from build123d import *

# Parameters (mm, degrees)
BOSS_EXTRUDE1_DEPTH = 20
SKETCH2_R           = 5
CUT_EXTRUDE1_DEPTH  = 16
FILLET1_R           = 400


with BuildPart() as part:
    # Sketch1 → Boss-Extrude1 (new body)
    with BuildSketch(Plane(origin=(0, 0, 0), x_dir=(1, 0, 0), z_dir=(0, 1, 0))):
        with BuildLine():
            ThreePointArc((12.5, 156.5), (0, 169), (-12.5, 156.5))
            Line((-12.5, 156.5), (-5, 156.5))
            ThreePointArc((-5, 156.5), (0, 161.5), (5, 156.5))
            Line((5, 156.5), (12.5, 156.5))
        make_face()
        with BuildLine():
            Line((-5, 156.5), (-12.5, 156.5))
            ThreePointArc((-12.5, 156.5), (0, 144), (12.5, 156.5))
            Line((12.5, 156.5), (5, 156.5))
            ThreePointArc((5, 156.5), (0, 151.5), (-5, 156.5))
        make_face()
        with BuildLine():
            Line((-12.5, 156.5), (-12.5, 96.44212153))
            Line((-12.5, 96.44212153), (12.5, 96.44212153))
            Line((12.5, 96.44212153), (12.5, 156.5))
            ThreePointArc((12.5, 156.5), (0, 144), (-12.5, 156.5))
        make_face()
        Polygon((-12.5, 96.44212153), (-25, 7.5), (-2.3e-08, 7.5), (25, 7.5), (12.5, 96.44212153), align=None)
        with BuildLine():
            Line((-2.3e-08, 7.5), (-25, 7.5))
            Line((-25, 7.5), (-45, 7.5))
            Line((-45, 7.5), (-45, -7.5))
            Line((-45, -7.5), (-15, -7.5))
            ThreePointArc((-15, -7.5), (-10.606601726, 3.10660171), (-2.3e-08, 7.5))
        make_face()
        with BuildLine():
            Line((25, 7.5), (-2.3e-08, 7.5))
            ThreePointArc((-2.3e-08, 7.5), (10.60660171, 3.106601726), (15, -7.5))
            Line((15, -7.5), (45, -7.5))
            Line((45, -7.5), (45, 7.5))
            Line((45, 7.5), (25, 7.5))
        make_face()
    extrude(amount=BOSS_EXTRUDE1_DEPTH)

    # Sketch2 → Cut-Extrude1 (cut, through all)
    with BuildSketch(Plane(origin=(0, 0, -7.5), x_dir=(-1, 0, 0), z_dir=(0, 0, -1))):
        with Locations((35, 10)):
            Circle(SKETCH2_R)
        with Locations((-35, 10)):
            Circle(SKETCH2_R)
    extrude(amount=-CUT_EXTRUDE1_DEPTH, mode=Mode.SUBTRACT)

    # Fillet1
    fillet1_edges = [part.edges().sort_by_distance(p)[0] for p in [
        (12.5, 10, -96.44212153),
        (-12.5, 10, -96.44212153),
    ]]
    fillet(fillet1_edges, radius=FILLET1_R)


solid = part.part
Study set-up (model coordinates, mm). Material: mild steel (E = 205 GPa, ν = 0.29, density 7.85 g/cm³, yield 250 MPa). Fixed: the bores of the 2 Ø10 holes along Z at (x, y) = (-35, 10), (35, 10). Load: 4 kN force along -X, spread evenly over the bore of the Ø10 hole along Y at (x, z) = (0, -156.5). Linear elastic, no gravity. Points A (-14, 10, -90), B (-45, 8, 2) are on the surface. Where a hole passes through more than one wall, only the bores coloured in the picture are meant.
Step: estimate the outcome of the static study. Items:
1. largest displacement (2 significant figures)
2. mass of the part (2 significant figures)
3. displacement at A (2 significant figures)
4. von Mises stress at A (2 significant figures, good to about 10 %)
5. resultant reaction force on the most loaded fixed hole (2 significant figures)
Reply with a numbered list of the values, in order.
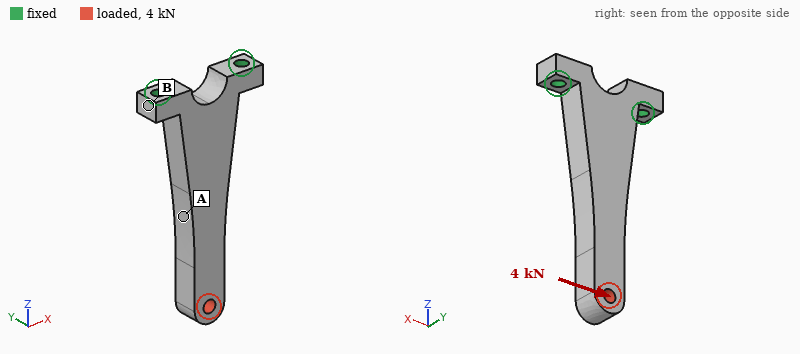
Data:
1. 0.39 mm
2. 930 g
3. 0.11 mm
4. 100 MPa
5. 12 kN
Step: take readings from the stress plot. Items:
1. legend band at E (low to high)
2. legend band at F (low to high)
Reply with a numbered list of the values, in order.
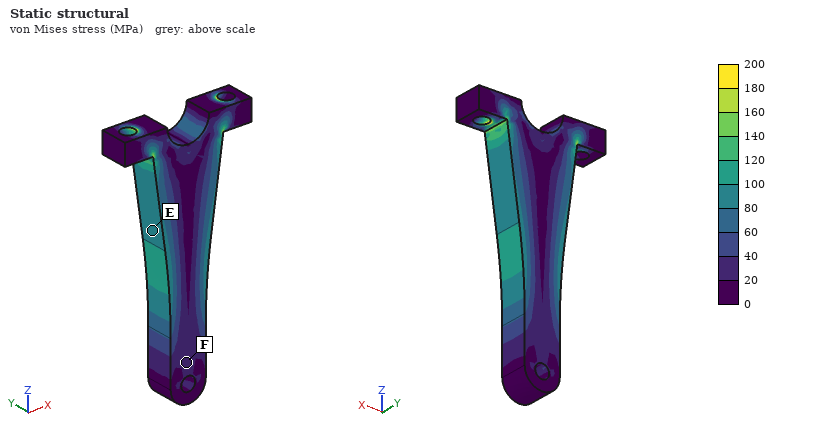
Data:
1. 80 to 100 MPa
2. 20 to 40 MPa
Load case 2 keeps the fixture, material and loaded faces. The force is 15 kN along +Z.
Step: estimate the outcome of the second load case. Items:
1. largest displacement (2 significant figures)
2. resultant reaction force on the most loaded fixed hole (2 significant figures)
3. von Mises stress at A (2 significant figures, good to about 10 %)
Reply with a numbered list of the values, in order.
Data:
1. 27 µm
2. 8.7 kN
3. 27 MPa
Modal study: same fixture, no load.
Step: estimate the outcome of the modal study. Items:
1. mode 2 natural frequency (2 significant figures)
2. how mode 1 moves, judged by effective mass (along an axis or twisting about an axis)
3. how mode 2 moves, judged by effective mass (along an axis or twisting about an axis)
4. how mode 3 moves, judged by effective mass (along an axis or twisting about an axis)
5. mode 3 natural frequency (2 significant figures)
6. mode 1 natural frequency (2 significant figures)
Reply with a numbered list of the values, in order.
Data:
1. 1300 Hz
2. along Y
3. along X
4. along Y
5. 3100 Hz
6. 560 Hz
